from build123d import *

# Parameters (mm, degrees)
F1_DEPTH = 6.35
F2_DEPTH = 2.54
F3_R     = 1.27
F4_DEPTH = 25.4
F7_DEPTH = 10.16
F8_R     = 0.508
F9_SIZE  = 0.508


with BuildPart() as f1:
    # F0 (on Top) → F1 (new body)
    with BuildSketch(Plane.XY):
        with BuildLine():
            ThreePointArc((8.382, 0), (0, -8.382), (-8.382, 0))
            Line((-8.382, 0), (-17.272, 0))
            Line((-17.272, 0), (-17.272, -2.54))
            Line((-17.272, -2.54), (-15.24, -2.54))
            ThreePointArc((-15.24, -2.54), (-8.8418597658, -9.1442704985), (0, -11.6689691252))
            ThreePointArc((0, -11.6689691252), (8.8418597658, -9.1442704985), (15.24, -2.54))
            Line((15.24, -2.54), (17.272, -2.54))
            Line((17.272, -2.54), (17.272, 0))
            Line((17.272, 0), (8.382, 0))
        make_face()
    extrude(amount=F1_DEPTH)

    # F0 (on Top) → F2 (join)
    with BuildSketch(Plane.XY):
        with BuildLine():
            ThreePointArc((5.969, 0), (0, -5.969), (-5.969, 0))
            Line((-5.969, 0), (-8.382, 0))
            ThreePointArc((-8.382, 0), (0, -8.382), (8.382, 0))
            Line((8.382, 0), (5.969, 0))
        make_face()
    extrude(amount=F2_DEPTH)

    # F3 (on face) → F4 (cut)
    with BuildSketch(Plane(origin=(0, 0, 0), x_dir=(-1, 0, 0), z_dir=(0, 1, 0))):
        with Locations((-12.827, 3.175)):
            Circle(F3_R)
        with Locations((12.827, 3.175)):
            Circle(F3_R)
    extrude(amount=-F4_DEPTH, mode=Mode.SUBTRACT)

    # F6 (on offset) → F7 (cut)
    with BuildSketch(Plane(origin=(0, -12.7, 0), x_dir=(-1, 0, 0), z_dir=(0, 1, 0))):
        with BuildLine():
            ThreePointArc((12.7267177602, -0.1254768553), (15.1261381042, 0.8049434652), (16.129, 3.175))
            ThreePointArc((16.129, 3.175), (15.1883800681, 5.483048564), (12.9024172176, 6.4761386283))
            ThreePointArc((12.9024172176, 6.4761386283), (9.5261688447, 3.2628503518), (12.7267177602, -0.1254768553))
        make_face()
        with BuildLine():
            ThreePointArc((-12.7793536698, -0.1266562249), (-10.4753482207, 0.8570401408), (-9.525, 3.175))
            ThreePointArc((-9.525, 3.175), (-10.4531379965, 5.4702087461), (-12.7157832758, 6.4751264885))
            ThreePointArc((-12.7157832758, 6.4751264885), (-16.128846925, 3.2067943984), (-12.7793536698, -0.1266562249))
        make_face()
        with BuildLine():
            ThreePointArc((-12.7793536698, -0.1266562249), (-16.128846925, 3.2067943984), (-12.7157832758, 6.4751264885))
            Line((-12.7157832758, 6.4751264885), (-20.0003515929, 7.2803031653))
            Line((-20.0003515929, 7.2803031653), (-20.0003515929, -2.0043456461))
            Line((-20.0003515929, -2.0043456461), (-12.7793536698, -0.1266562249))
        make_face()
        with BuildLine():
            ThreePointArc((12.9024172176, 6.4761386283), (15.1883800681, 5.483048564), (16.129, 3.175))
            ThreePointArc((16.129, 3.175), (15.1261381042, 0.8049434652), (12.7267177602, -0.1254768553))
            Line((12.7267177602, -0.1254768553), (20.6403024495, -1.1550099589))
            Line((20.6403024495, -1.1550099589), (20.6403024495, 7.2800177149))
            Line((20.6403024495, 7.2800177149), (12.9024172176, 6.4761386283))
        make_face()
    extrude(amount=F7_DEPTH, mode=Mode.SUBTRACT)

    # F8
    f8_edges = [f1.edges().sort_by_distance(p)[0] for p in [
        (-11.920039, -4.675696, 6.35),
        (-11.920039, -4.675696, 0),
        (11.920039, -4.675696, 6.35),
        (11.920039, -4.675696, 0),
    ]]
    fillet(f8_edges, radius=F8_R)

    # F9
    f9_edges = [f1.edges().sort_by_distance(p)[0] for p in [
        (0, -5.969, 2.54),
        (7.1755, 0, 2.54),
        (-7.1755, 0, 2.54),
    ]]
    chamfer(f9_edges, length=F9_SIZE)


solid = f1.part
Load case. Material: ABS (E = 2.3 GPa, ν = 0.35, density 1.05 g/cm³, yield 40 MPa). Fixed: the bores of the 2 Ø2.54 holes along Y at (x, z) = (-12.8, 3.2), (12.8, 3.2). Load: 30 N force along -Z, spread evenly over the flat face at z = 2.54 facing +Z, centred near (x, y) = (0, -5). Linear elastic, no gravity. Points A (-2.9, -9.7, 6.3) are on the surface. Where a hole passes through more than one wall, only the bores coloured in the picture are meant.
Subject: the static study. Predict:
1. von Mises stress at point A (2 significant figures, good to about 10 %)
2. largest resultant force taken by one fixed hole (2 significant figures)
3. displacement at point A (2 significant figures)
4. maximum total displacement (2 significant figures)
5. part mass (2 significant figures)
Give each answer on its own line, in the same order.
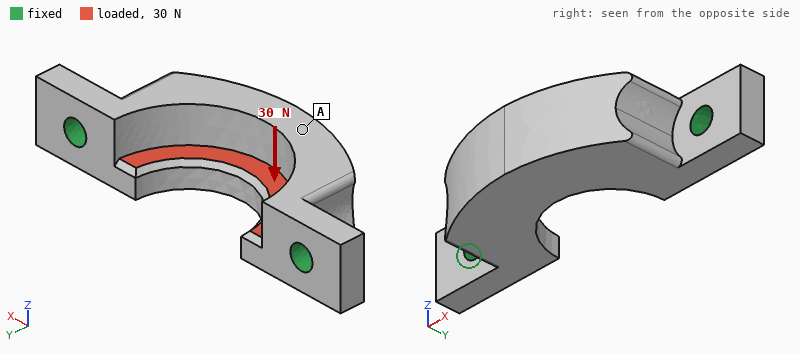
1.6 MPa
15 N
68 µm
81 µm
1.0 g
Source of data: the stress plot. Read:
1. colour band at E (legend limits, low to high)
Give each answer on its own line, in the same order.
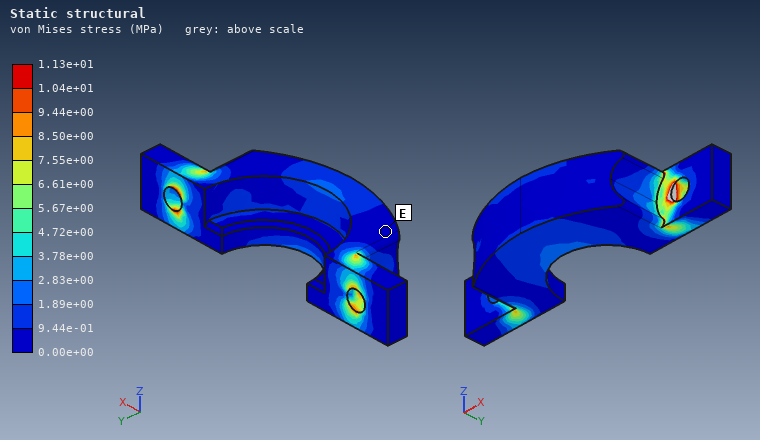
0.00e+00 to 9.44e-01 MPa
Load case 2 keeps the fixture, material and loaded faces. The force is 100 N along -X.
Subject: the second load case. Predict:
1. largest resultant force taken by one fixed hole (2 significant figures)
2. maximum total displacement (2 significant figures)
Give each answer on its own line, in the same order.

52 N
34 µm
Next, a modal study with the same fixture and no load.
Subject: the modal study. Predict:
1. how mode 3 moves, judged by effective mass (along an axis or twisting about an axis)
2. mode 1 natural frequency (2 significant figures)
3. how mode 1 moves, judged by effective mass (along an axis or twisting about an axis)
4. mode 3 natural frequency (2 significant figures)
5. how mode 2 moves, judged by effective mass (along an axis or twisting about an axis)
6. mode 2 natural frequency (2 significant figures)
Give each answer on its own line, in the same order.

along Y
3400 Hz
along Z
10 kHz
along X
8300 Hz
